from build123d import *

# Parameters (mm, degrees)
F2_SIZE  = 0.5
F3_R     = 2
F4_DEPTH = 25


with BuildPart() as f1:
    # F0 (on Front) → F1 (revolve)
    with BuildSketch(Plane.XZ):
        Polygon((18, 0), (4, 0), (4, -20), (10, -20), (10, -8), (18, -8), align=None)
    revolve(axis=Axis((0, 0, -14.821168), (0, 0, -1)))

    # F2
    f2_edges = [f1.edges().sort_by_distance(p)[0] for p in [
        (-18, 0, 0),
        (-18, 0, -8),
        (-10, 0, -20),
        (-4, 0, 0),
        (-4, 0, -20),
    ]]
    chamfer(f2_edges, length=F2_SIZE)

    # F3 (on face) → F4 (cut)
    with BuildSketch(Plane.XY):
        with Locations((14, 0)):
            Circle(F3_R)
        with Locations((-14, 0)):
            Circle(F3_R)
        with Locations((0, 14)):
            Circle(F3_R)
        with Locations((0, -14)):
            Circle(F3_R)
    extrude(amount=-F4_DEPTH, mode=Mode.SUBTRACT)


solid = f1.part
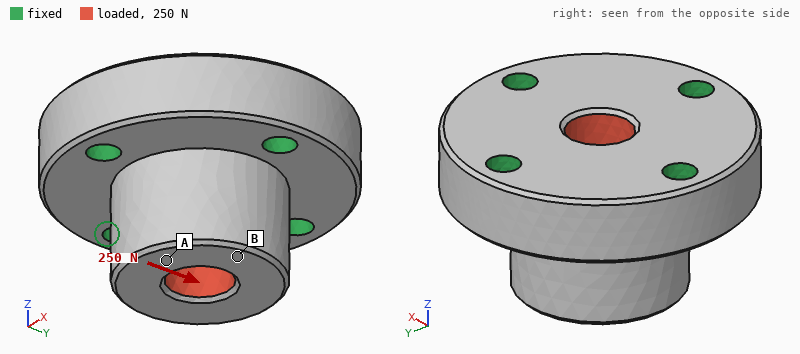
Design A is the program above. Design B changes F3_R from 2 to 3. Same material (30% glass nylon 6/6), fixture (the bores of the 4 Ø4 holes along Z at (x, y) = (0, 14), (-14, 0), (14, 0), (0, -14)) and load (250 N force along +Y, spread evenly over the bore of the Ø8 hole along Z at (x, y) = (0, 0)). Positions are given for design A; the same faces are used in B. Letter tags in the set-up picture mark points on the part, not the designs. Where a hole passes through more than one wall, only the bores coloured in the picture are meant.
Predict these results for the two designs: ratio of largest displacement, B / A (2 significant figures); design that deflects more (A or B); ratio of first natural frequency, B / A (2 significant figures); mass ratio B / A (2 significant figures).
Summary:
0.86
A
1.1
0.95
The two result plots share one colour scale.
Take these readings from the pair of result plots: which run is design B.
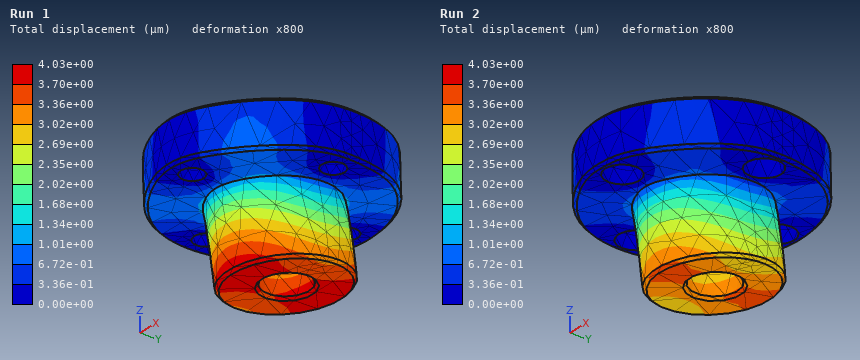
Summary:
Run 2
